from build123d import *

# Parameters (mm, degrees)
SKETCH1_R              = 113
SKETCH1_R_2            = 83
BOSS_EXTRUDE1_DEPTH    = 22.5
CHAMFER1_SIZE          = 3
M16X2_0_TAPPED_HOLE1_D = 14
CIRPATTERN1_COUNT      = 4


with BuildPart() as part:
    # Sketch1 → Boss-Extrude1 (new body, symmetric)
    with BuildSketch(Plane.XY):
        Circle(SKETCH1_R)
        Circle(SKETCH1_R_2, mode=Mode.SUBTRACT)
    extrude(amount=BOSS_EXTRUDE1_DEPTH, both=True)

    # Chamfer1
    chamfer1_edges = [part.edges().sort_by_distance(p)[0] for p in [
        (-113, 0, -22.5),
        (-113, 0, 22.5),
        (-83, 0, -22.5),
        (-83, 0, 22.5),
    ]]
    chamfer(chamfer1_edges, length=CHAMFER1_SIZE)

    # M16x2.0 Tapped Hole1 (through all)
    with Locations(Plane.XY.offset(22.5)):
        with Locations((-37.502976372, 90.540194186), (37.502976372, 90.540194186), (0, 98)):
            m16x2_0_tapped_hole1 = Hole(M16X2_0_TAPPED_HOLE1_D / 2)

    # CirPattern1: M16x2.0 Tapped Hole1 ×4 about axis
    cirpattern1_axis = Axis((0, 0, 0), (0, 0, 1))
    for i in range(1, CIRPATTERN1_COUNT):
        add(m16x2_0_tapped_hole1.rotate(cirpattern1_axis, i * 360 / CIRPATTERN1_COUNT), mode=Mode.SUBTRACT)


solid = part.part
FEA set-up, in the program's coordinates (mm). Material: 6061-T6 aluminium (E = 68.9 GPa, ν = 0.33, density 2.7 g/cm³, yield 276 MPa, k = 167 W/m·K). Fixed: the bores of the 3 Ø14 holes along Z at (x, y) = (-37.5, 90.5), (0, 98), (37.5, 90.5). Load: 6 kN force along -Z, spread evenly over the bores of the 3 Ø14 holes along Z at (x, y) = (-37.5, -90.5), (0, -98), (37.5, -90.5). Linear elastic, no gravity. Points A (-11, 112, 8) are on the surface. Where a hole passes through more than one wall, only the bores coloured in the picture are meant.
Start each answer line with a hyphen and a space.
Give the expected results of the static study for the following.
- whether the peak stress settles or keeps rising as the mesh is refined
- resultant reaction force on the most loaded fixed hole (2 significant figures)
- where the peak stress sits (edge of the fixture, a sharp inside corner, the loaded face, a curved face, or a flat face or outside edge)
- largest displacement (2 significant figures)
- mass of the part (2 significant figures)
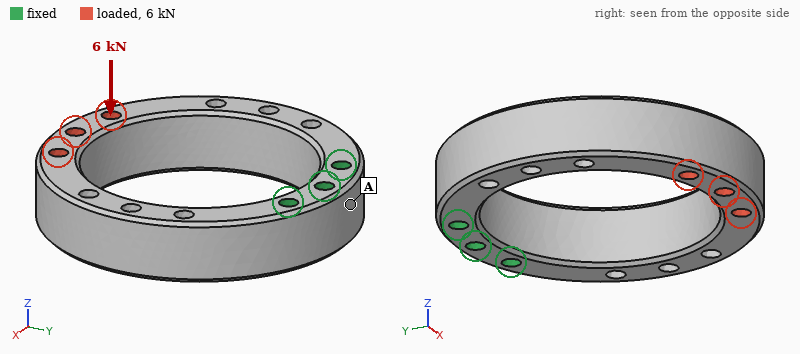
- keeps rising
- 3.2 kN
- edge of the fixture
- 1.1 mm
- 2.0 kg
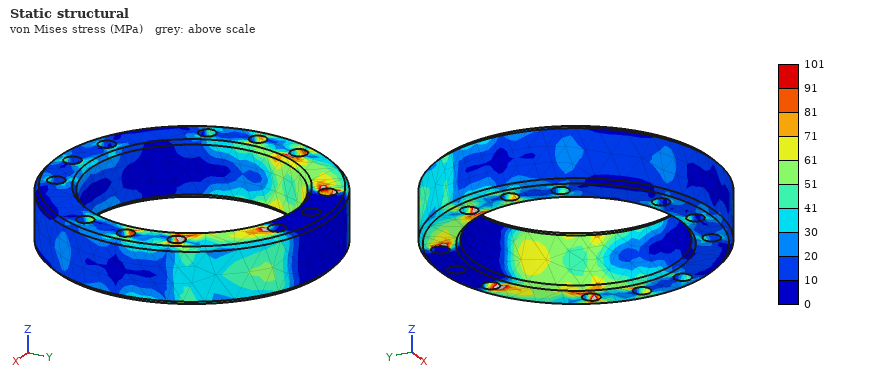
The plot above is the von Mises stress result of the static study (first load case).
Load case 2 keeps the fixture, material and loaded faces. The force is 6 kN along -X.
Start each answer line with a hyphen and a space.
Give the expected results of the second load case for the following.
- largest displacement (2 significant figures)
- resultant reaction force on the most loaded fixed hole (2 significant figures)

- 0.49 mm
- 6.7 kN
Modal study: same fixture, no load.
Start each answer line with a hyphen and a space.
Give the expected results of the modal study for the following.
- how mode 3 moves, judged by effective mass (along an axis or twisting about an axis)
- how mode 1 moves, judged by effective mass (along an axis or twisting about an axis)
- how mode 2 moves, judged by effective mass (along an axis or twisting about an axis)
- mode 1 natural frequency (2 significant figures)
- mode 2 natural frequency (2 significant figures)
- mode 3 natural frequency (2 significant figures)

- twisting about Y
- along Z
- along X
- 500 Hz
- 600 Hz
- 1300 Hz
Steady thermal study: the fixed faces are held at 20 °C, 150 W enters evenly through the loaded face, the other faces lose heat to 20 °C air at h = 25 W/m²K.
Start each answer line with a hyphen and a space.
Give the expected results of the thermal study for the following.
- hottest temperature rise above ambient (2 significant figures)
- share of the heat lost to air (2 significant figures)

- 65 K
- 44 %
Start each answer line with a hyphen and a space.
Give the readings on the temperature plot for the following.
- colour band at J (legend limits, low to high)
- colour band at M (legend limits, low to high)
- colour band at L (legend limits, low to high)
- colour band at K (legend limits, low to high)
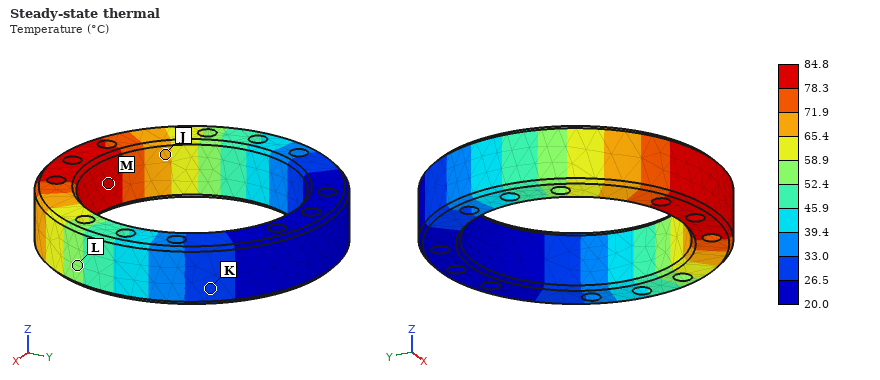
- 65.4 to 71.9 °C
- 78.3 to 84.8 °C
- 52.4 to 58.9 °C
- 26.5 to 33.0 °C
